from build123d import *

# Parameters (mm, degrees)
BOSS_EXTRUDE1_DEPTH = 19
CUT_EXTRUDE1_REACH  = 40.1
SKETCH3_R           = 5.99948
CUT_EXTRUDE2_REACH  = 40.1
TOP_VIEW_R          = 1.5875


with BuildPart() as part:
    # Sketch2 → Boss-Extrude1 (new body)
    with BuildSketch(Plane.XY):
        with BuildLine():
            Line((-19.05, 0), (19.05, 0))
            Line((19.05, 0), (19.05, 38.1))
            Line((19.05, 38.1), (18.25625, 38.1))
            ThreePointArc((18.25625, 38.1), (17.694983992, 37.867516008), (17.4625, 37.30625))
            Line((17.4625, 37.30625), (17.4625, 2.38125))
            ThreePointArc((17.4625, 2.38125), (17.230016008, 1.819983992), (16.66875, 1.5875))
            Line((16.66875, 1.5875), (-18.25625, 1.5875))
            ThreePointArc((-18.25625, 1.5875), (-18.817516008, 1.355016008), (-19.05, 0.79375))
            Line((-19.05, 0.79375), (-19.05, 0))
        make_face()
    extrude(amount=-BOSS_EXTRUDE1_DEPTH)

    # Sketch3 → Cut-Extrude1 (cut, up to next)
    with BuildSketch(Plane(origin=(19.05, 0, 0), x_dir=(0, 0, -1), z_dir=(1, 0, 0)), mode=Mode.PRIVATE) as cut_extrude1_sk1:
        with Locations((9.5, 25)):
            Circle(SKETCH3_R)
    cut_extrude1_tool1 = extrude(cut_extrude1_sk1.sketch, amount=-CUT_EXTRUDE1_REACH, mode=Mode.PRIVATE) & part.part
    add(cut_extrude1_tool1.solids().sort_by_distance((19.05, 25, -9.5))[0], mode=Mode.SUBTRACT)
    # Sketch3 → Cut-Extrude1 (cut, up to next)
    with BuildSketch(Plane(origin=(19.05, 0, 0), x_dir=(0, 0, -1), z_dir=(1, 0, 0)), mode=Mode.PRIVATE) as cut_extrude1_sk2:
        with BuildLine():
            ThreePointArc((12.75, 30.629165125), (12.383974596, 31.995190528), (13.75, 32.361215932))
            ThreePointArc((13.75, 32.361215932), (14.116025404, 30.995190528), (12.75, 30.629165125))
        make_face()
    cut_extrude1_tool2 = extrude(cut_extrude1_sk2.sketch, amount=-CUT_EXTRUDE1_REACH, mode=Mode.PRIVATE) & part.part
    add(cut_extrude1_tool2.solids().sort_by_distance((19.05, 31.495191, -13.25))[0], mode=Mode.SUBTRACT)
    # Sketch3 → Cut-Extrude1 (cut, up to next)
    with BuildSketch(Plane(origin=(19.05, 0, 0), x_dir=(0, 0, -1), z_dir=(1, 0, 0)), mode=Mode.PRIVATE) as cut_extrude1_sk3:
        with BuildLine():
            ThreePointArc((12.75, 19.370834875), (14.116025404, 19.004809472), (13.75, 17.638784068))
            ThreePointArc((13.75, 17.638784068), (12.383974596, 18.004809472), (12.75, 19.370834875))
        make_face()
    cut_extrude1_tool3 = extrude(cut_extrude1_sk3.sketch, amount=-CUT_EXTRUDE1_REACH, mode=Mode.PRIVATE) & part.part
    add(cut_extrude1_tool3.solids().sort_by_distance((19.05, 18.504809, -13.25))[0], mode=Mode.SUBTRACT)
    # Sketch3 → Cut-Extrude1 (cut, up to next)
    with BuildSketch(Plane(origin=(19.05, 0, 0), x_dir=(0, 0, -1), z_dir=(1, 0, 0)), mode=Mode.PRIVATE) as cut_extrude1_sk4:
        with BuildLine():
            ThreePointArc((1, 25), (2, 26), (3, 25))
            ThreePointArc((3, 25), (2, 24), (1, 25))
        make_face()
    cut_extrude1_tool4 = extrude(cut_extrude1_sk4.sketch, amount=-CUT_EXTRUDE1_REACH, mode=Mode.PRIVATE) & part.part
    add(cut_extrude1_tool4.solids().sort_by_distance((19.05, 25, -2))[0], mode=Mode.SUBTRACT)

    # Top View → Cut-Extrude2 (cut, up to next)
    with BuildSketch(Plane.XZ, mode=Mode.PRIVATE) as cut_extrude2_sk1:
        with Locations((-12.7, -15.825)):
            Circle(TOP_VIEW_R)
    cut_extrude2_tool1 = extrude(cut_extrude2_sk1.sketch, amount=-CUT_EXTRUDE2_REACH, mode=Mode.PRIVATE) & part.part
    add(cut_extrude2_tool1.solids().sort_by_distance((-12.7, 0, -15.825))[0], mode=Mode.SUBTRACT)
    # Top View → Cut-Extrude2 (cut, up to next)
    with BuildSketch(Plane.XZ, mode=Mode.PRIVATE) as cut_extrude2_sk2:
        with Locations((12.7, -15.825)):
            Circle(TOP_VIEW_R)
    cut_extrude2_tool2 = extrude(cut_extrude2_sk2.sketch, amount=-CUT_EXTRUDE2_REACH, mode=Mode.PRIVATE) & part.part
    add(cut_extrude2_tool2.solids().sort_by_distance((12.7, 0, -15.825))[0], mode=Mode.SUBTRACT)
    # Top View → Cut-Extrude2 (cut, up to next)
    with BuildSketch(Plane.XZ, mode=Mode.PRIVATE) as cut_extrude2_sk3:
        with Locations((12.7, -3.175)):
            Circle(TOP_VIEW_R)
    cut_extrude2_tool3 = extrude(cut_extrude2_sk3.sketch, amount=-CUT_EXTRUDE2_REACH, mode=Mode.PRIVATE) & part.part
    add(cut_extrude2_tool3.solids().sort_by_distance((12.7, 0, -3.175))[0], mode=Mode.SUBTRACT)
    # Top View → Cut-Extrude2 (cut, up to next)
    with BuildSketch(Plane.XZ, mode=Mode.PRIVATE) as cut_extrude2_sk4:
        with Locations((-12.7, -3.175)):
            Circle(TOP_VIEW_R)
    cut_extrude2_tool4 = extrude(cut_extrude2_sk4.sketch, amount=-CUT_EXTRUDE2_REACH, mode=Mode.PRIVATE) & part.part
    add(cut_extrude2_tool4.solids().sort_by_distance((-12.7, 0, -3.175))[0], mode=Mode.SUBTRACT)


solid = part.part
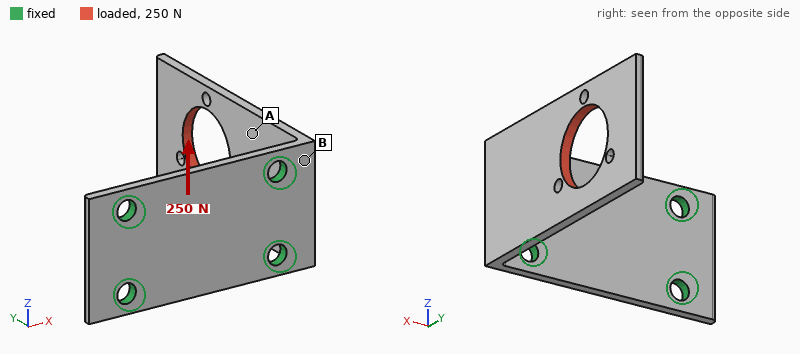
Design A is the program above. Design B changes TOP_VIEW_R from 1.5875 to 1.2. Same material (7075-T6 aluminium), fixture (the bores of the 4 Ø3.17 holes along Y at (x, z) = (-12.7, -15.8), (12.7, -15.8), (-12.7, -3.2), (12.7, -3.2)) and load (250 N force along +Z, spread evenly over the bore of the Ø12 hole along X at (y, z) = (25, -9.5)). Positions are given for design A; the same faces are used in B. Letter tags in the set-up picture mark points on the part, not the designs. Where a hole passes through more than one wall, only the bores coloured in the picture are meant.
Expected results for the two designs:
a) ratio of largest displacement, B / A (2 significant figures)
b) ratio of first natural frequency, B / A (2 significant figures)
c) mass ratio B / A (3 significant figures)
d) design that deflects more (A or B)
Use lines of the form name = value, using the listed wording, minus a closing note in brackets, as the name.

ratio of largest displacement, B / A = 1.2
ratio of first natural frequency, B / A = 0.98
mass ratio B / A = 1.01
design that deflects more = B
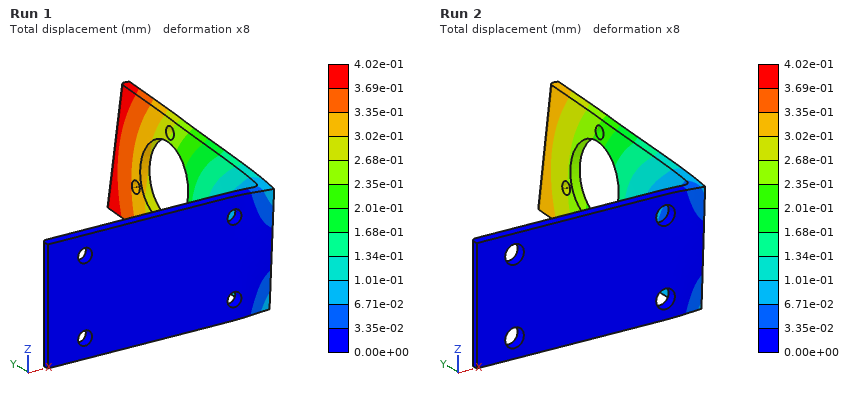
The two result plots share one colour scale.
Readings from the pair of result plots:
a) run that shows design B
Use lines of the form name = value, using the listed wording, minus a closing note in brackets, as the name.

run that shows design B = Run 1
